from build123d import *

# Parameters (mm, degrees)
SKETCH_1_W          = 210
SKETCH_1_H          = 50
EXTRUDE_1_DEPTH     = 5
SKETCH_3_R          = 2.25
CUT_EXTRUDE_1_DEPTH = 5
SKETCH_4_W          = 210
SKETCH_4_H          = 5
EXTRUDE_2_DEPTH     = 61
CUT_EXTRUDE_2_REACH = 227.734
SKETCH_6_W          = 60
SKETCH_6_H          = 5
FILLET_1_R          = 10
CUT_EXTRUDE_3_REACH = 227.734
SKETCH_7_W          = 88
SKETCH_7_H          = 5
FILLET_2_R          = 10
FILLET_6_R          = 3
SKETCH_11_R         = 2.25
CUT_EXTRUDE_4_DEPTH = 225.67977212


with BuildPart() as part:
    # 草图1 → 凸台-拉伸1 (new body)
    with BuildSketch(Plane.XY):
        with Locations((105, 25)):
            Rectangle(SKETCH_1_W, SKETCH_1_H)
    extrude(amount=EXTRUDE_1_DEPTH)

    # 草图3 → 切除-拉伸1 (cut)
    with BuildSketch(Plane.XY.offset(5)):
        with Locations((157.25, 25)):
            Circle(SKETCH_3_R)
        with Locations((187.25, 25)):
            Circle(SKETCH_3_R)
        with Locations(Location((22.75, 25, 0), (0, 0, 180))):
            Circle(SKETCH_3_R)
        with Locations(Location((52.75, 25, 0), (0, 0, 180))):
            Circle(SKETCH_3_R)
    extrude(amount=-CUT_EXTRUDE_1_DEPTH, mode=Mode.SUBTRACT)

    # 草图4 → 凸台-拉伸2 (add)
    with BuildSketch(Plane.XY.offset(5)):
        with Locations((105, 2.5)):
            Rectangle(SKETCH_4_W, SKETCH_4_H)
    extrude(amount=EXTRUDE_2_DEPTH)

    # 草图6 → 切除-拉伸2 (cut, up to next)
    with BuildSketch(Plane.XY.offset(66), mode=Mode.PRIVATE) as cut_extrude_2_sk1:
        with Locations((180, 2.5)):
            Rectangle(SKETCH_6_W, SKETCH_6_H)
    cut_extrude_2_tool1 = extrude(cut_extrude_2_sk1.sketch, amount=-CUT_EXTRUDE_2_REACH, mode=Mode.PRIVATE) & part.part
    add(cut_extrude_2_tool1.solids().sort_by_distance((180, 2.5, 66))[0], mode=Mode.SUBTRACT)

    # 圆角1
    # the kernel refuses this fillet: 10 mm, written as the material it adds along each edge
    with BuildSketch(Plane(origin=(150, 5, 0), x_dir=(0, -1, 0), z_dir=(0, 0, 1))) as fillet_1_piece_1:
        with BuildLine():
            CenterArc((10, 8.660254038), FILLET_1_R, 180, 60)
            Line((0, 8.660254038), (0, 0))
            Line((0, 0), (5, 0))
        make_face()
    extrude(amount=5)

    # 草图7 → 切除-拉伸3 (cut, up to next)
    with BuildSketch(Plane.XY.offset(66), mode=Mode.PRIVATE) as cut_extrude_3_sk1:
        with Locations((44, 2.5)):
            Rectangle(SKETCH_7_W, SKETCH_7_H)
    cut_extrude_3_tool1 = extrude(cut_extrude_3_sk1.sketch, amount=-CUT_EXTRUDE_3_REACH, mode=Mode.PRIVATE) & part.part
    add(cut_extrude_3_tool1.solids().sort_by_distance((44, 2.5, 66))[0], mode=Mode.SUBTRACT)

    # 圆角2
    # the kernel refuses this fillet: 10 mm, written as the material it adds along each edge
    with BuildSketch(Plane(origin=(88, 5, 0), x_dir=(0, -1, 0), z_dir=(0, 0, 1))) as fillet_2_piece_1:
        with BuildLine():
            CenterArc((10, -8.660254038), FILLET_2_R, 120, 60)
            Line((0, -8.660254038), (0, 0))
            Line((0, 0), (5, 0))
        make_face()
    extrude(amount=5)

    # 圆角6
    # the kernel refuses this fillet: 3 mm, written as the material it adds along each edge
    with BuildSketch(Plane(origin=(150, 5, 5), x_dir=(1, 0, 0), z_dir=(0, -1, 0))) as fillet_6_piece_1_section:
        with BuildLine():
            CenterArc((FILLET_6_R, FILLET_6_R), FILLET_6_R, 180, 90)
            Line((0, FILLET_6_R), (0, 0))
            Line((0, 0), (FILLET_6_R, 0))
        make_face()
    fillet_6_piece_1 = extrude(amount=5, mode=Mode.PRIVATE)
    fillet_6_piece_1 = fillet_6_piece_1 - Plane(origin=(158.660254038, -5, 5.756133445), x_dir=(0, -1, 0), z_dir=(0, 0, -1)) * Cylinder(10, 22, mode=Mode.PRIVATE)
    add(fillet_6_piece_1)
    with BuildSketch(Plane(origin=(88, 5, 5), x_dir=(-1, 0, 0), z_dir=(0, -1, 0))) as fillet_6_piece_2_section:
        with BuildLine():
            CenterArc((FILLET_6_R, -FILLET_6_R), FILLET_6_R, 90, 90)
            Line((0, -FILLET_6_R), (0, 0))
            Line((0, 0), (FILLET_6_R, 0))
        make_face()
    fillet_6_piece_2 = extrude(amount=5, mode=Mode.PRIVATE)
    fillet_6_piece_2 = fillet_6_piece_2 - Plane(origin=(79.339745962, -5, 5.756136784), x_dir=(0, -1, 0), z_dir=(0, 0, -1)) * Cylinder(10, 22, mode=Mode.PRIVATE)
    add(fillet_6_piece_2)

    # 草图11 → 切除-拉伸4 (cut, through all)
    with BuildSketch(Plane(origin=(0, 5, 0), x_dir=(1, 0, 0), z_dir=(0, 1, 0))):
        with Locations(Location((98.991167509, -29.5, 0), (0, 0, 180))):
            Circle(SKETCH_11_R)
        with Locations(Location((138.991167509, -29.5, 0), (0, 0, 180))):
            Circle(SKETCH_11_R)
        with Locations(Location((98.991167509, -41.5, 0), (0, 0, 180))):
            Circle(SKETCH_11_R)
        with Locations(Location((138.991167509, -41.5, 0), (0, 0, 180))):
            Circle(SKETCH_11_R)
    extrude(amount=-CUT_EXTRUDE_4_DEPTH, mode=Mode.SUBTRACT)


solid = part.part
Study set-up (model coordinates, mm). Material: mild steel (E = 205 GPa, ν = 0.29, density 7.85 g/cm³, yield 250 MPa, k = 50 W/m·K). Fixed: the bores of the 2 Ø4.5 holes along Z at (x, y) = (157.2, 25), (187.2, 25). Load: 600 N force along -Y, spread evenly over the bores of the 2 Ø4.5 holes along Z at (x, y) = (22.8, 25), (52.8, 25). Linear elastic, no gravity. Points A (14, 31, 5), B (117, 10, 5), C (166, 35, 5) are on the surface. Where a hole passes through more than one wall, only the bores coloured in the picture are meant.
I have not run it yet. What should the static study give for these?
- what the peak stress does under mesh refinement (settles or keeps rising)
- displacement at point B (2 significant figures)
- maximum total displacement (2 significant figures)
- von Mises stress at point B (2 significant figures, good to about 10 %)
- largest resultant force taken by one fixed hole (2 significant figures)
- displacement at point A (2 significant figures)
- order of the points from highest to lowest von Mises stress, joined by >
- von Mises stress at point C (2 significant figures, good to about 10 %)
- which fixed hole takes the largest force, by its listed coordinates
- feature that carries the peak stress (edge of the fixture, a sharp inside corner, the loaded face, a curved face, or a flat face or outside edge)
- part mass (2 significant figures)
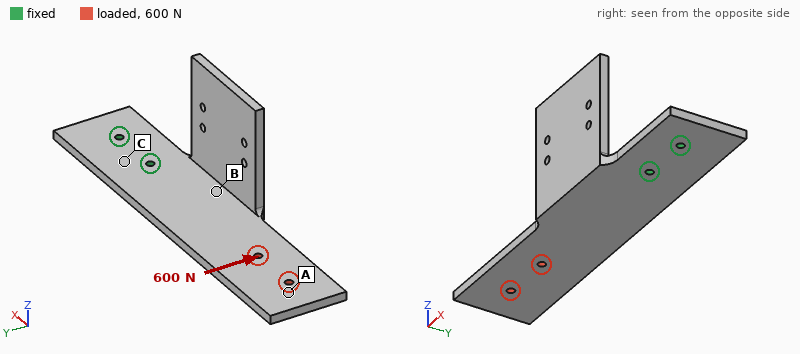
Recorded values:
keeps rising
19 µm
98 µm
8.8 MPa
2.7 kN
87 µm
C > B > A
23 MPa
(157.2, 25)
edge of the fixture
530 g
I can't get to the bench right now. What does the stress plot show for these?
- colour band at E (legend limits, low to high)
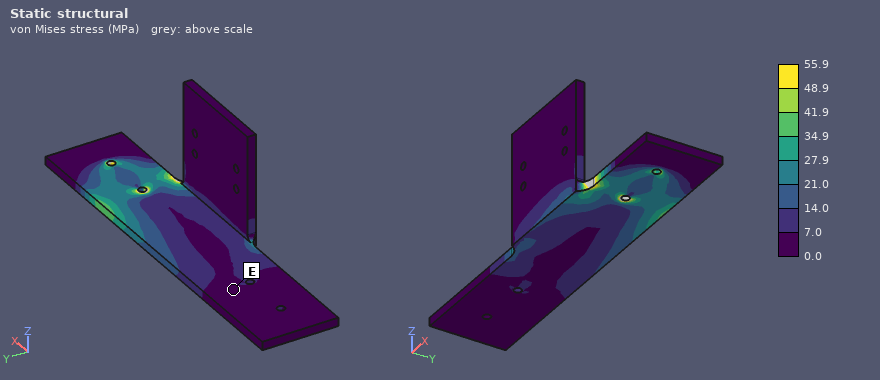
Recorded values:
0.0 to 7.0 MPa
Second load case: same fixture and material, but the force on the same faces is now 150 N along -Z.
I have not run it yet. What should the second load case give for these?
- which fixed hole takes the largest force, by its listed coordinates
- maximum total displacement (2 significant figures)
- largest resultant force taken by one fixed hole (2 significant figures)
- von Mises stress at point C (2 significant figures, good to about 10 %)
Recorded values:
(157.2, 25)
0.83 mm
420 N
17 MPa
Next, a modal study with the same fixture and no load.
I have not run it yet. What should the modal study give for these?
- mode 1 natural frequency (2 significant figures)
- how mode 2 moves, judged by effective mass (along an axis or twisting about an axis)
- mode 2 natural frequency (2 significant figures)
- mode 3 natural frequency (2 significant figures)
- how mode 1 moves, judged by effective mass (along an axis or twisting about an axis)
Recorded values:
200 Hz
along Y
500 Hz
800 Hz
along Z
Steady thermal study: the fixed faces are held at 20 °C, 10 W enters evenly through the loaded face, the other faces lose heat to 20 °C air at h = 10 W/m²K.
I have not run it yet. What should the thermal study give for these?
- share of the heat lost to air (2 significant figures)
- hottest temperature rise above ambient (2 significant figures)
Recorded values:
61 %
58 K
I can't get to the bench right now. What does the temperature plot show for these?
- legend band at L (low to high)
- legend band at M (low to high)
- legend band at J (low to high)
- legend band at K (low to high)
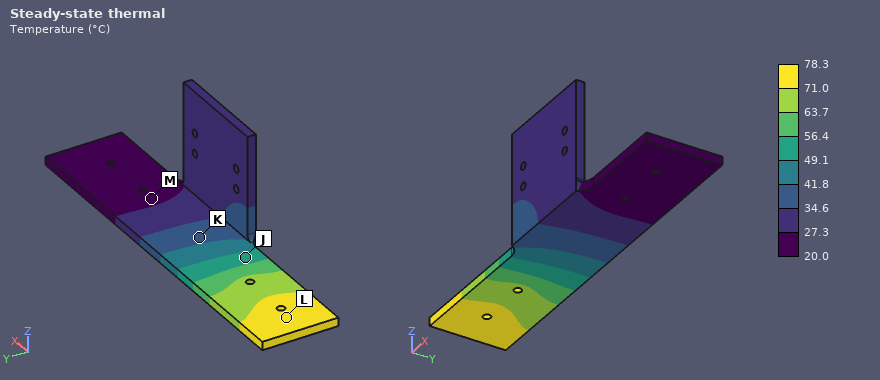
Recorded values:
71.0 to 78.3 °C
20.0 to 27.3 °C
49.1 to 56.4 °C
34.6 to 41.8 °C
